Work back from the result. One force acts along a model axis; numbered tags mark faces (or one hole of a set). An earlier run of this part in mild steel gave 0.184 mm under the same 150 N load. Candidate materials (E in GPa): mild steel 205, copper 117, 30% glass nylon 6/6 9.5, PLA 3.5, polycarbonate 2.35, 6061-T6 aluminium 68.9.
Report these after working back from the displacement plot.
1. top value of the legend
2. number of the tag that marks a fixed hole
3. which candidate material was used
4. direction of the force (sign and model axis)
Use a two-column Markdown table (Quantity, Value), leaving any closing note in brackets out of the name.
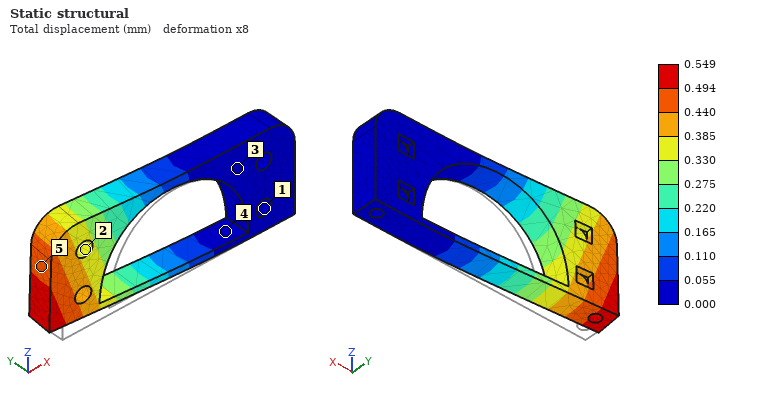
| Quantity | Value |
|---|---|
| top value of the legend | 0.549 mm |
| number of the tag that marks a fixed hole | 1 |
| which candidate material was used | 6061-T6 aluminium |
| direction of the force | +Y |
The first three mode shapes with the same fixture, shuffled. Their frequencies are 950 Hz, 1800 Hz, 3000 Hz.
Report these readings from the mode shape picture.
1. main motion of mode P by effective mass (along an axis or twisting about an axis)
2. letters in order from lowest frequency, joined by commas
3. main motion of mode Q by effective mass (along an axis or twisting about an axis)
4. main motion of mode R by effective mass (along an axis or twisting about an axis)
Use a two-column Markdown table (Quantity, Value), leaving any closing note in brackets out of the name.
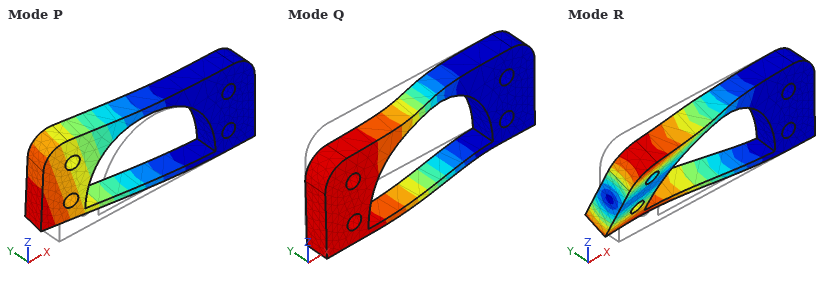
| Quantity | Value |
|---|---|
| main motion of mode P by effective mass | along Y |
| letters in order from lowest frequency, joined by commas | P, Q, R |
| main motion of mode Q by effective mass | along Z |
| main motion of mode R by effective mass | twisting about X |
